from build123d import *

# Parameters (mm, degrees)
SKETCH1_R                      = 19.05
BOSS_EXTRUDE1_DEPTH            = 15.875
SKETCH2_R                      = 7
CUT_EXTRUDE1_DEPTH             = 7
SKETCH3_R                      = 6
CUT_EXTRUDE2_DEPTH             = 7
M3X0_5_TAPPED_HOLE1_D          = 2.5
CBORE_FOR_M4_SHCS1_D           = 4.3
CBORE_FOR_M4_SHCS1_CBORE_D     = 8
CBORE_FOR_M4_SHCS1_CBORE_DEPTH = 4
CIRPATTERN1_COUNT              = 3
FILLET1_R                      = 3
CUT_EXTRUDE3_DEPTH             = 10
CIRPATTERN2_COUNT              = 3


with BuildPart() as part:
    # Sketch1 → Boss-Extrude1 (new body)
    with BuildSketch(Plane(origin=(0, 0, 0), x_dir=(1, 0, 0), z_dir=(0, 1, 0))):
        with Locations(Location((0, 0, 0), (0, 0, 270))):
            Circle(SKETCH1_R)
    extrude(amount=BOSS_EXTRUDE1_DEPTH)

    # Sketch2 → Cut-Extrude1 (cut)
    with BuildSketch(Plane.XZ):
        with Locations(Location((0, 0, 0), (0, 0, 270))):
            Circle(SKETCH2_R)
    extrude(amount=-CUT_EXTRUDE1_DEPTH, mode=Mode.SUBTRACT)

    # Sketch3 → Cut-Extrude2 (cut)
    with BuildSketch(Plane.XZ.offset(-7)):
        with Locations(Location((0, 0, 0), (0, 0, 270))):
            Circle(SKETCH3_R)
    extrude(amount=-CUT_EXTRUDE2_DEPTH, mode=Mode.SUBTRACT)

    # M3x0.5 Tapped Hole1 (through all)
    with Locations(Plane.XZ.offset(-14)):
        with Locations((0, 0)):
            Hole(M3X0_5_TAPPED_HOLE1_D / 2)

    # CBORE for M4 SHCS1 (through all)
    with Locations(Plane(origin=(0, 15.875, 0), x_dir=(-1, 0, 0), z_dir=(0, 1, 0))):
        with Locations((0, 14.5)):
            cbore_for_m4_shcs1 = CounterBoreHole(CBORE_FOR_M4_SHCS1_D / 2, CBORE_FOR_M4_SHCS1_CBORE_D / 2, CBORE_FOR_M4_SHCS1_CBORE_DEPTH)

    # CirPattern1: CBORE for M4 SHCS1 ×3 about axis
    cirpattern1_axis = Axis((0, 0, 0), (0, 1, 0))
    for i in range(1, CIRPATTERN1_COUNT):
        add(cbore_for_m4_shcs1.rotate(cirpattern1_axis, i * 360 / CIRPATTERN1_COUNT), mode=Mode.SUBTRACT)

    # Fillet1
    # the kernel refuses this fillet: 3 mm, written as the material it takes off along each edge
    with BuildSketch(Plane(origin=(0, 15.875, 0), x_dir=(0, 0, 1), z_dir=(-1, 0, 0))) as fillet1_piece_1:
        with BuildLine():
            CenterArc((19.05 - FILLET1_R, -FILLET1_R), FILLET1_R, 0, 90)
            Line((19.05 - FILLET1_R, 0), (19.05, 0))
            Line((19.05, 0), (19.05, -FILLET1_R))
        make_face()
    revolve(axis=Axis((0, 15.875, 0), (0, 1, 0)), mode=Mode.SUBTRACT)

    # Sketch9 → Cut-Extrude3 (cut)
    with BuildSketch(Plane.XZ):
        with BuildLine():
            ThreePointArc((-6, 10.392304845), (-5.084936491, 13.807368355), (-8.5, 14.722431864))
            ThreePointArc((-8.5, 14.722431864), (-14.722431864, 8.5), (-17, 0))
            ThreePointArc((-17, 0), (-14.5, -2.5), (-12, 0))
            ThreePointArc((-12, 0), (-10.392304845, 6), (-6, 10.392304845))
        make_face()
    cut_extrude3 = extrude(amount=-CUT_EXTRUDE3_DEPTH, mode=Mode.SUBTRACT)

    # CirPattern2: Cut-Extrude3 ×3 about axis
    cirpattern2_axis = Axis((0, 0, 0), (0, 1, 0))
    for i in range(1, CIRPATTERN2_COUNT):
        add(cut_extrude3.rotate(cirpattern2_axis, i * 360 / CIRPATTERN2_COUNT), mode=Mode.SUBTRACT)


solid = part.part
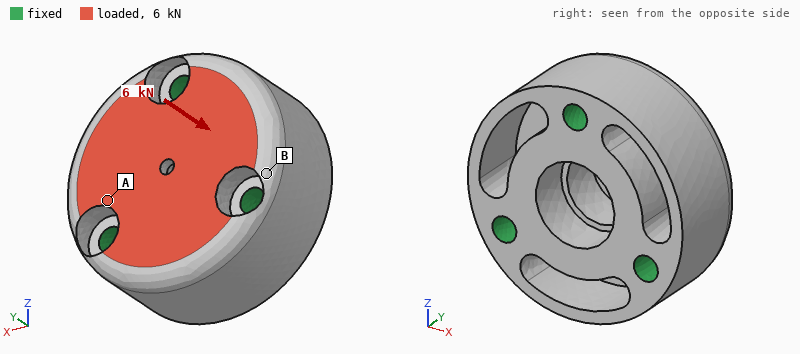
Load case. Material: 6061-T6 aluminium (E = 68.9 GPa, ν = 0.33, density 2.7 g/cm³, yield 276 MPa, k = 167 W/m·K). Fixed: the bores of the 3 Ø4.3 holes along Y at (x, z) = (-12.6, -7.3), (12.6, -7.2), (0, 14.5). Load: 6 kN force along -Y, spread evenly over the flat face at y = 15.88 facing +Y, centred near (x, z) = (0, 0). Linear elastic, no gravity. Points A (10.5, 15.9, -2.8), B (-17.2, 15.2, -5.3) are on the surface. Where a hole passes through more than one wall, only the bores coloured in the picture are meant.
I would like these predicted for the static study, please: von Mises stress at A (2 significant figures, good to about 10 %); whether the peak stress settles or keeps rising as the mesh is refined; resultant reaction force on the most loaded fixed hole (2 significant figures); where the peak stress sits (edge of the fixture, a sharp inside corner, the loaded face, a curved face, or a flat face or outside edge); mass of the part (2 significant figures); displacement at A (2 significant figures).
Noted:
13 MPa
keeps rising
2.1 kN
a sharp inside corner
32 g
3.1 µm
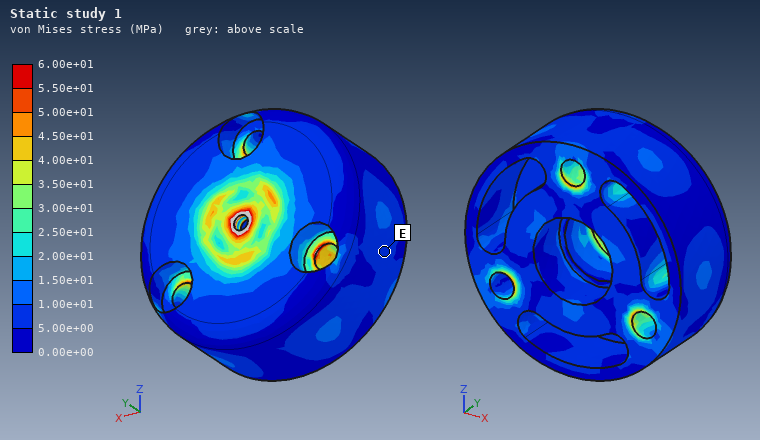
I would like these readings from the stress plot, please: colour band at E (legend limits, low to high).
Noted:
5.00e+00 to 1.00e+01 MPa
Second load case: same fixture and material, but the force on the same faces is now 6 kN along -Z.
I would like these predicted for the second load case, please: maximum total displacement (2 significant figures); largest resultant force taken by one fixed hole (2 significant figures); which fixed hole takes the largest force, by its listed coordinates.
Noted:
11 µm
2.6 kN
(0, 14.5)
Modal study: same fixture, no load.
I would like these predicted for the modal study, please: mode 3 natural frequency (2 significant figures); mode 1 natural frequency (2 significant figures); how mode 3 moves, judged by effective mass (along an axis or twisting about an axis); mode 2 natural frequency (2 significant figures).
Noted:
37 kHz
33 kHz
along Y
33 kHz
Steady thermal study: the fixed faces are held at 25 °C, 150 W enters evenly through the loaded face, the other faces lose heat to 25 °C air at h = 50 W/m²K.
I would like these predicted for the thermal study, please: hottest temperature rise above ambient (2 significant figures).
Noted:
25 K
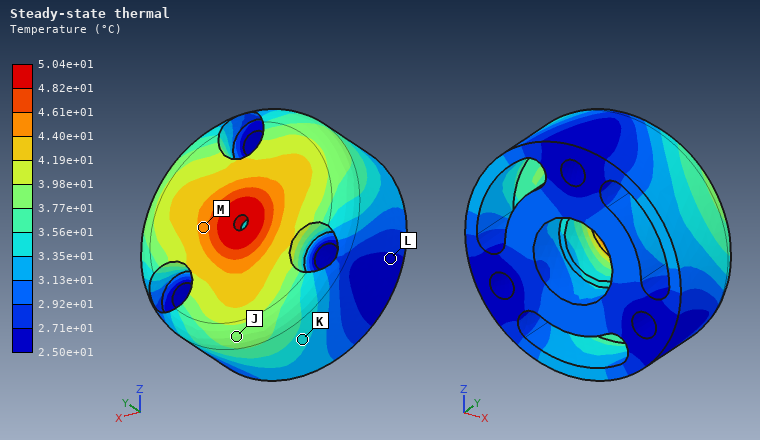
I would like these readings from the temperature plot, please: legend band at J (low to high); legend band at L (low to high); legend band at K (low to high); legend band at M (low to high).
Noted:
3.77e+01 to 3.98e+01 °C
2.50e+01 to 2.71e+01 °C
3.35e+01 to 3.56e+01 °C
4.40e+01 to 4.61e+01 °C
